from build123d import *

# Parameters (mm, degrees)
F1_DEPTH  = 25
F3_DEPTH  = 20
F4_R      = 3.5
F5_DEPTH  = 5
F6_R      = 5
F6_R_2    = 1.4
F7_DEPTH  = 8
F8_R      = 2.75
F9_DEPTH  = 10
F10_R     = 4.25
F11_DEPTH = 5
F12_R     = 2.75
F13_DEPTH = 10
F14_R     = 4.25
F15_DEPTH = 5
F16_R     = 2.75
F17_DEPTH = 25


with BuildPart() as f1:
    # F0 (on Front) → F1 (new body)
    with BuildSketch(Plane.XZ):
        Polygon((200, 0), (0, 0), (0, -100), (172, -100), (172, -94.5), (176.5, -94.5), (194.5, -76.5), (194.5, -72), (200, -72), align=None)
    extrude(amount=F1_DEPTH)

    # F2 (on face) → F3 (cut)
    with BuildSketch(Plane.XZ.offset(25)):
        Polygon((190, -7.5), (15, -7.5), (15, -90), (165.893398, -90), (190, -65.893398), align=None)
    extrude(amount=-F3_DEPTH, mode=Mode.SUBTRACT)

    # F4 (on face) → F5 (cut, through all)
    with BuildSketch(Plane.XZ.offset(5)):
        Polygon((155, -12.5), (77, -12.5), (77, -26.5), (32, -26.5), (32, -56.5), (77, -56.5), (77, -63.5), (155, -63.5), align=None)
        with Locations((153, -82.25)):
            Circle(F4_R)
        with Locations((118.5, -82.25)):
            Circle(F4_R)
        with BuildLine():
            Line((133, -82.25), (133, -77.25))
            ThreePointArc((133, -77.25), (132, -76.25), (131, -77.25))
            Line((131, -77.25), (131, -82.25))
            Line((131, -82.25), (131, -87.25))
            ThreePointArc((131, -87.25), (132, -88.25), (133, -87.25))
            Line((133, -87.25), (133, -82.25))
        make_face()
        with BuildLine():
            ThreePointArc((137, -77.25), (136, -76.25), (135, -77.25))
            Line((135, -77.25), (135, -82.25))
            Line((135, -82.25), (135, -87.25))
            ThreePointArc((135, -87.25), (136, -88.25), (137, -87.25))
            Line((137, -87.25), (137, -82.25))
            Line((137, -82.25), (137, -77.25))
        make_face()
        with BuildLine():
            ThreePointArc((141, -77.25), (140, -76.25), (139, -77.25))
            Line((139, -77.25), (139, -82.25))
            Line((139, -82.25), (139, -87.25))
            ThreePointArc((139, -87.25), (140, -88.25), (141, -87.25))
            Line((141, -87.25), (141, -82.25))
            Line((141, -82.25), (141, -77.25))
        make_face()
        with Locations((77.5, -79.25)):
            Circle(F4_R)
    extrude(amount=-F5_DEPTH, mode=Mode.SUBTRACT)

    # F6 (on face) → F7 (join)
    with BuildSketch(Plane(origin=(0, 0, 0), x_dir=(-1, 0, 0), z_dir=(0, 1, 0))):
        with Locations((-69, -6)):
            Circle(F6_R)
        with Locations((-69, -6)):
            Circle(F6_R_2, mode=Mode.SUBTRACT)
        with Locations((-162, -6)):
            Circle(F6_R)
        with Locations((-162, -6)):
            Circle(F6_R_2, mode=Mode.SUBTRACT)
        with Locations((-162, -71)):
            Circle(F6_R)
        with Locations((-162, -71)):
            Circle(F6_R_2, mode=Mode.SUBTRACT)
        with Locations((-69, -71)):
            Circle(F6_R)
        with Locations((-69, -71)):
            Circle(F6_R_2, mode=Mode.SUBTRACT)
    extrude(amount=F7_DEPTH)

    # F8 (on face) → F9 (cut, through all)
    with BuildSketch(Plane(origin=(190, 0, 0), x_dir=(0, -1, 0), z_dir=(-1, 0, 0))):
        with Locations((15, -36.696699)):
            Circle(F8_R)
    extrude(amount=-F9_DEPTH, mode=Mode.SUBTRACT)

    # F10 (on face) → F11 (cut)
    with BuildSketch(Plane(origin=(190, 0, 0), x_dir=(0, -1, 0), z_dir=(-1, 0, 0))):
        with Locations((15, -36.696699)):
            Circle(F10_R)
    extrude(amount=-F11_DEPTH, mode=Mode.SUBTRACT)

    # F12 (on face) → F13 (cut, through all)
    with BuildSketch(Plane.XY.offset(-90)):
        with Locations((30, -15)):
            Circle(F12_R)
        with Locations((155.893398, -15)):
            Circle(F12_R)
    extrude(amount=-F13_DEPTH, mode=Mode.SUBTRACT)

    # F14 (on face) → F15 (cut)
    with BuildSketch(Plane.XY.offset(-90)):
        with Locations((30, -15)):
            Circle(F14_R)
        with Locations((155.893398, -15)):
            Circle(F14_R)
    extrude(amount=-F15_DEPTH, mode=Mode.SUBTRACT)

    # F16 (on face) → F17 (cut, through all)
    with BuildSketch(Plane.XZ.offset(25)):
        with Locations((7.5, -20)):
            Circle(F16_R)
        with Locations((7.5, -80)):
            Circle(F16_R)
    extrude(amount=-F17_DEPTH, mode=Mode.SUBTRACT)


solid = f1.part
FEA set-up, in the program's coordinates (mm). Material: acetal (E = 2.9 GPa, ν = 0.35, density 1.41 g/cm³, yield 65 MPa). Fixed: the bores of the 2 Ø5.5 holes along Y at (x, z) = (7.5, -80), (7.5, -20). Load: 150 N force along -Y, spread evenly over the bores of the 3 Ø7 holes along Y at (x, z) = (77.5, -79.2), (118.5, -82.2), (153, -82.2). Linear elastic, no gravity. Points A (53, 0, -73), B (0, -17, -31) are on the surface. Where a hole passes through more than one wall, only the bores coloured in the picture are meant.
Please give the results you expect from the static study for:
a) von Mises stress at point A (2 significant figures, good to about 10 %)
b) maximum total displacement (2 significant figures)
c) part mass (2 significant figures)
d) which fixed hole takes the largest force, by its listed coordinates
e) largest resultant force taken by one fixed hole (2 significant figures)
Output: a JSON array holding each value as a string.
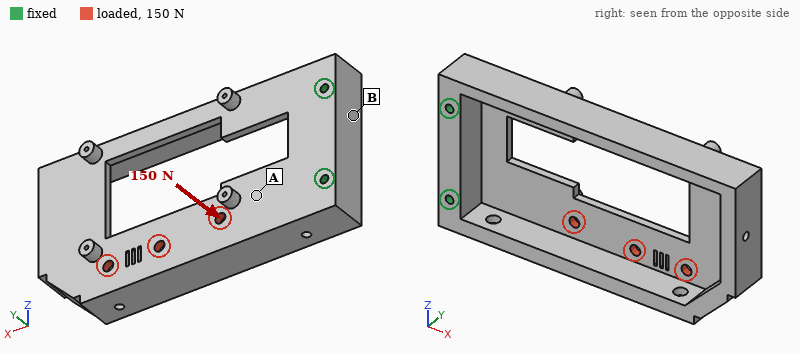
["2.5 MPa", "2.3 mm", "250 g", "(7.5, -80)", "130 N"]
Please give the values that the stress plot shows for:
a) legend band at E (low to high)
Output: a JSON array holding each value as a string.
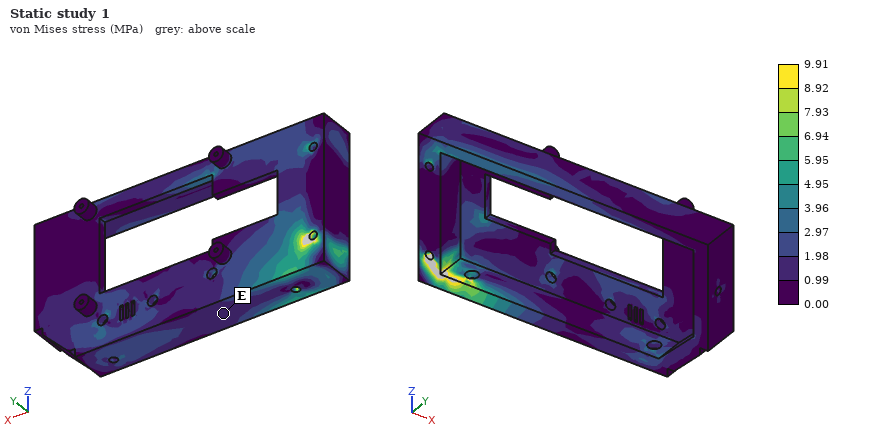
["0.99 to 1.98 MPa"]
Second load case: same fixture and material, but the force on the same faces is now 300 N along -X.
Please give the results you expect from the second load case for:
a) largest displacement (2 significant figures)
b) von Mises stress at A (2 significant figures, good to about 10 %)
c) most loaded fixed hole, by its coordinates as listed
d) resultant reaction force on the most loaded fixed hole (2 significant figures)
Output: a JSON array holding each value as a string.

["0.32 mm", "1.4 MPa", "(7.5, -80)", "290 N"]
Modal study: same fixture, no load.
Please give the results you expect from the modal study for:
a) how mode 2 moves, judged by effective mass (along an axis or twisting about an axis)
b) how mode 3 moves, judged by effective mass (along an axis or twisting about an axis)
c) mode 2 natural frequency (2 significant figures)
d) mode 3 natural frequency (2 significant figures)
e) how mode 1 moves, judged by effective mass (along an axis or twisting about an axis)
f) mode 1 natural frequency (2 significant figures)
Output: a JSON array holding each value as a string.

["along Z", "along Z", "170 Hz", "290 Hz", "along Y", "110 Hz"]
